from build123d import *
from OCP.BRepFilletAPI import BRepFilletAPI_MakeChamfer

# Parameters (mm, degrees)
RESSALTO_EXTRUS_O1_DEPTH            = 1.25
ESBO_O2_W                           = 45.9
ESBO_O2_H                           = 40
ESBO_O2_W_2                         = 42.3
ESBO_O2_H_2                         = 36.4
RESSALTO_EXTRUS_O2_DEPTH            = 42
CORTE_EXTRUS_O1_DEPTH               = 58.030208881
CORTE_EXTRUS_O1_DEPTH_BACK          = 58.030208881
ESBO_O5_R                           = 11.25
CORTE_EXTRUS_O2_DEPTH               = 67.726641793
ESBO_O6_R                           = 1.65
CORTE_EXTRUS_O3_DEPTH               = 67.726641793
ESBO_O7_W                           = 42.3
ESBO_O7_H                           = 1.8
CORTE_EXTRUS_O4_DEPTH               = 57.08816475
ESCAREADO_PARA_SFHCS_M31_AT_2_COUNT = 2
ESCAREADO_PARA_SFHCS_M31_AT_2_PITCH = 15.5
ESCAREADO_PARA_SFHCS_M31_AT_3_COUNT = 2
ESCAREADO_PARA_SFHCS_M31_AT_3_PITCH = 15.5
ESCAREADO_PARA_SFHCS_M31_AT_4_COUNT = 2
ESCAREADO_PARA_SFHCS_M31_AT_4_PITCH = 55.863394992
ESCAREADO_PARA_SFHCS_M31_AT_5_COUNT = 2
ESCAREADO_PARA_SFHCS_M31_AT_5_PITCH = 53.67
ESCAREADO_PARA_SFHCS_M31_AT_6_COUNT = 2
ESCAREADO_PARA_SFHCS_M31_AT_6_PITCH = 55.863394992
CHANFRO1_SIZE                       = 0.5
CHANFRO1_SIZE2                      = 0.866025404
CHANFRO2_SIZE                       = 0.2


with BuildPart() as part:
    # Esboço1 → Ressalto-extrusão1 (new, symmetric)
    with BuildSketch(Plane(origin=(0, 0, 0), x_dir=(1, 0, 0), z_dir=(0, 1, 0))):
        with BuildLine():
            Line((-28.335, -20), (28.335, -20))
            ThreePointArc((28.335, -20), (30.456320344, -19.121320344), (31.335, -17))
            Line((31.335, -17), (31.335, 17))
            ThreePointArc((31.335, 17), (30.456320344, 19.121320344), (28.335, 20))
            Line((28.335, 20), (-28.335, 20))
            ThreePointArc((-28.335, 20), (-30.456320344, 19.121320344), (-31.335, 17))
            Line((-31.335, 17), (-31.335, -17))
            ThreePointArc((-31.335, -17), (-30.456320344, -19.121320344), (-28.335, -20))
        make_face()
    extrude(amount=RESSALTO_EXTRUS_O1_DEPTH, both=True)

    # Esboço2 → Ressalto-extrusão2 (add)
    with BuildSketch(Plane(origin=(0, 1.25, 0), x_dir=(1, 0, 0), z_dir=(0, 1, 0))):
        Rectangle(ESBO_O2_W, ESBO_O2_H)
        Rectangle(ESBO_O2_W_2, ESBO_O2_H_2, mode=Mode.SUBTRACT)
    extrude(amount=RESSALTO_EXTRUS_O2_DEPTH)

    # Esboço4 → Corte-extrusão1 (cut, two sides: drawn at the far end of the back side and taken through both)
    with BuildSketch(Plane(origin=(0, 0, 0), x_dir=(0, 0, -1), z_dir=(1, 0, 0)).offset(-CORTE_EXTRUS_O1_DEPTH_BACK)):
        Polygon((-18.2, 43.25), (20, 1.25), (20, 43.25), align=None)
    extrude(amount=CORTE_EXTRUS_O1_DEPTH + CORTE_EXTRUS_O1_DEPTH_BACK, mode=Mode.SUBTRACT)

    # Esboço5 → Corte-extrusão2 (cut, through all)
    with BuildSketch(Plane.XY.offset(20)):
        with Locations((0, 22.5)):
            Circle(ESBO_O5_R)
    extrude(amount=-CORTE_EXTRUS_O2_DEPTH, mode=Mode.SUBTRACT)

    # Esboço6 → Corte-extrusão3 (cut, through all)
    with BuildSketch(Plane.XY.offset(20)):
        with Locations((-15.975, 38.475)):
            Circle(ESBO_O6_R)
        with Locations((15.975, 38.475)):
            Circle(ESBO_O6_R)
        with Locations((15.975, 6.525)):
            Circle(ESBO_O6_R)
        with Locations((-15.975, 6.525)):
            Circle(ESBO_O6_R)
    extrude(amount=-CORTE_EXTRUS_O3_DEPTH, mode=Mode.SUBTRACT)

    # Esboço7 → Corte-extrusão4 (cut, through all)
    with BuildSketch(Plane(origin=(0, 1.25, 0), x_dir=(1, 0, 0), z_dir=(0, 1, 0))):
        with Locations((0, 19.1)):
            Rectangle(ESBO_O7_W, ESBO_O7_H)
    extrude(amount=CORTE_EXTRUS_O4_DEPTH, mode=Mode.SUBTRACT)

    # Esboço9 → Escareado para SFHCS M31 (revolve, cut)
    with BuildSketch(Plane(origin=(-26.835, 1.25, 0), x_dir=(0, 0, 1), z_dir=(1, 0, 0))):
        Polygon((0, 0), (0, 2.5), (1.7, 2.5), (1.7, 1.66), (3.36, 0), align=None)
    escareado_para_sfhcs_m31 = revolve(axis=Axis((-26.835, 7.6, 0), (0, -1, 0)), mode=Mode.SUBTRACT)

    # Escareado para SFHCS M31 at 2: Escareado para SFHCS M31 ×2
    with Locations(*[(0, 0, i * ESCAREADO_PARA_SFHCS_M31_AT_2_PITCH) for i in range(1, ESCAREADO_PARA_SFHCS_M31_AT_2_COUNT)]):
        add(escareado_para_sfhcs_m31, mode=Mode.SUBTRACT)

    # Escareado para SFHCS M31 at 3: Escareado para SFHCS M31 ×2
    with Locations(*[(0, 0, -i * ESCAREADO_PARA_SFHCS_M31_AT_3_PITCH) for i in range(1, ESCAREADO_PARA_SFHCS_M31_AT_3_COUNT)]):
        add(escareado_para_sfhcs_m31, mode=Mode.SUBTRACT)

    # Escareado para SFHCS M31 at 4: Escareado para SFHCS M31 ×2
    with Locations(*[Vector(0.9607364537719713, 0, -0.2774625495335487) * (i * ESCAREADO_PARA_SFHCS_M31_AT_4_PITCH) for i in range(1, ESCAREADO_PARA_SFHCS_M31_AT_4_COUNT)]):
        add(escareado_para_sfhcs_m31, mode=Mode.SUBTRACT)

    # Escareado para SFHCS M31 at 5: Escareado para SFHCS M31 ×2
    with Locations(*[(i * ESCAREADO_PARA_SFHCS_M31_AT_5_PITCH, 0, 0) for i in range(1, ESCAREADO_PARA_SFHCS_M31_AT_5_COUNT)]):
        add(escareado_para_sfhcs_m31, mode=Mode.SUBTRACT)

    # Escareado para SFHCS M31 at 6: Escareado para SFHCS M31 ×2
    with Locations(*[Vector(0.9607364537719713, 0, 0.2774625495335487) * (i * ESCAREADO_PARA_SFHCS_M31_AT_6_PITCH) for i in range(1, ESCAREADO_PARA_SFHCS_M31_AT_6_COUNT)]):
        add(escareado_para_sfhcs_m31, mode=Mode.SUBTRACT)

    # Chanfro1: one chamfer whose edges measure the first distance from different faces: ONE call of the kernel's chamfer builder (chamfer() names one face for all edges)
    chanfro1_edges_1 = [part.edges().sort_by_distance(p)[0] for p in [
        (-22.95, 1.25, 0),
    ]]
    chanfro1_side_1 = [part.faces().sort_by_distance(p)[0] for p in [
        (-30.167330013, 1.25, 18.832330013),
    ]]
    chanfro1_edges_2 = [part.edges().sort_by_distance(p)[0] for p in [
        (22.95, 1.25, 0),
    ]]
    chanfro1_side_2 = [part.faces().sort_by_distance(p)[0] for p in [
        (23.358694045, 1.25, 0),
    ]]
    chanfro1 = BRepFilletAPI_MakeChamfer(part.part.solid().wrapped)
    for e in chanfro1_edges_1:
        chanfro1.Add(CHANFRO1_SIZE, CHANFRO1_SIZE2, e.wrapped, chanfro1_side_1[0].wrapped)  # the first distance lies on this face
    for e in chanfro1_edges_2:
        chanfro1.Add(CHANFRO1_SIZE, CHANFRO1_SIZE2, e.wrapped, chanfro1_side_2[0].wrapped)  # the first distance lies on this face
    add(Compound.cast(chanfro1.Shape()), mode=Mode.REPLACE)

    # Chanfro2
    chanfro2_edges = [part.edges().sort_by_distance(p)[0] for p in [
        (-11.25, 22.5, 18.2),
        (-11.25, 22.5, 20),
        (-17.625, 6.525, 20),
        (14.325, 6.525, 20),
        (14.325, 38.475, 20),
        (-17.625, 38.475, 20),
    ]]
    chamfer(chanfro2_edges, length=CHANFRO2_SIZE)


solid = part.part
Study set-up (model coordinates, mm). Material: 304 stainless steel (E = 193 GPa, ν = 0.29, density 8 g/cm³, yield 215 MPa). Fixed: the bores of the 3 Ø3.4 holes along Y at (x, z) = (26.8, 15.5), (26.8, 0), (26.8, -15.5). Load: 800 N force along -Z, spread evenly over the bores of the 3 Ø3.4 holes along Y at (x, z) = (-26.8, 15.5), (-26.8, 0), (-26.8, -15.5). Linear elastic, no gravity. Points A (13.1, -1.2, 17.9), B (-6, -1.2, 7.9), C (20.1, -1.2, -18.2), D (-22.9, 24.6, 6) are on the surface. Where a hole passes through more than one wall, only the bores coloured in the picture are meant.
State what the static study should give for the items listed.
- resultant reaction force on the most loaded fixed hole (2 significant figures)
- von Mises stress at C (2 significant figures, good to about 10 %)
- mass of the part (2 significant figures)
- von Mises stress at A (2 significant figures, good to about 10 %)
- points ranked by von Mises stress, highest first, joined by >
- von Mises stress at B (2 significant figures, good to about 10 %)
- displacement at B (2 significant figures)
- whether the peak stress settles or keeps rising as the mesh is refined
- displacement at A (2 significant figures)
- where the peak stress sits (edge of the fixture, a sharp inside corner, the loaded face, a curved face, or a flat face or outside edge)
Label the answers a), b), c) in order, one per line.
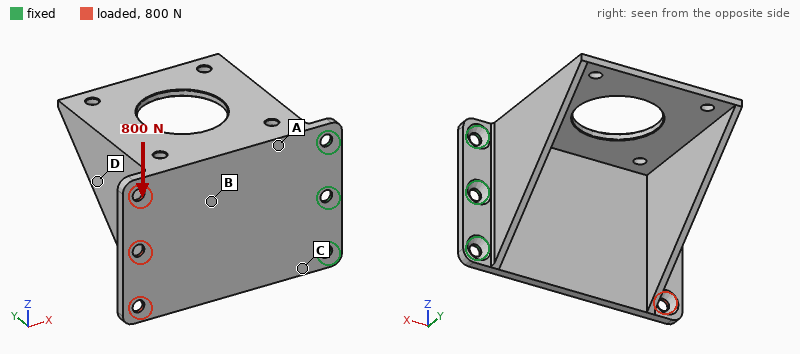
a) 1.4 kN
b) 68 MPa
c) 93 g
d) 39 MPa
e) C > A > B > D
f) 27 MPa
g) 18 µm
h) keeps rising
i) 13 µm
j) edge of the fixture
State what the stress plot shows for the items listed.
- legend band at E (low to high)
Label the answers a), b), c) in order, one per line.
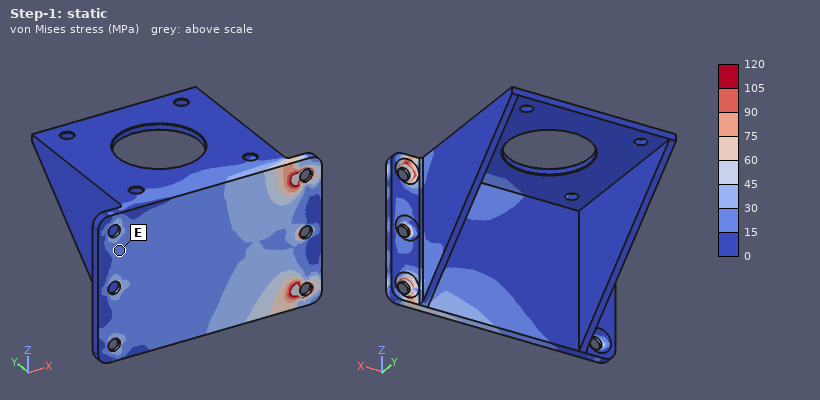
a) 15 to 30 MPa
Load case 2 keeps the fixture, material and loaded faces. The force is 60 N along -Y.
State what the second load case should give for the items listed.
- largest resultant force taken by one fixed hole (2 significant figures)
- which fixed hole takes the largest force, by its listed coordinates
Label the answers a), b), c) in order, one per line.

a) 41 N
b) (26.8, 0)
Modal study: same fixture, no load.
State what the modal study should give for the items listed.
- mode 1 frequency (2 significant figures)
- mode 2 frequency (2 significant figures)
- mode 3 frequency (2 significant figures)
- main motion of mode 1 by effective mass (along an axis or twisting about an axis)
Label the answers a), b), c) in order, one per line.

a) 420 Hz
b) 1100 Hz
c) 3200 Hz
d) along Y
